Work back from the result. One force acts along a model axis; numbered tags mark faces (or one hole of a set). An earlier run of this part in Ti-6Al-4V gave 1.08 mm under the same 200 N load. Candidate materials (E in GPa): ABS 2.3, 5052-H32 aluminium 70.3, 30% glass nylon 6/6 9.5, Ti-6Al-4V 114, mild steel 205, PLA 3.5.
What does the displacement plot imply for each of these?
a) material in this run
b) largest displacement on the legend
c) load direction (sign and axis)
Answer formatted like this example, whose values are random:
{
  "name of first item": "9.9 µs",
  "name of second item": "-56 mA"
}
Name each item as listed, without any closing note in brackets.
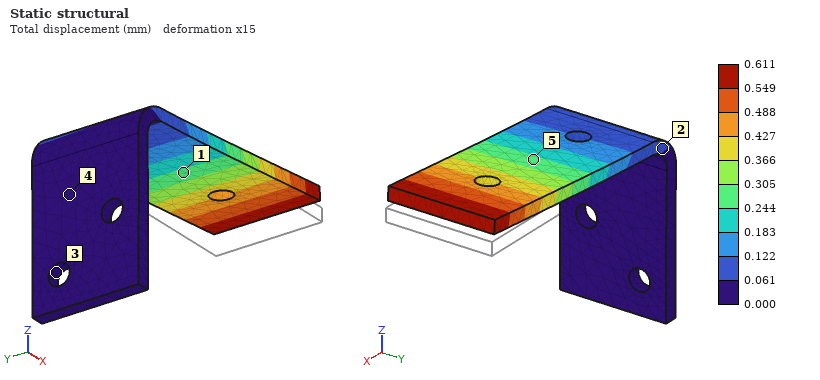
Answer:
{
  "material in this run": "mild steel",
  "largest displacement on the legend": "0.611 mm",
  "load direction": "+Z"
}
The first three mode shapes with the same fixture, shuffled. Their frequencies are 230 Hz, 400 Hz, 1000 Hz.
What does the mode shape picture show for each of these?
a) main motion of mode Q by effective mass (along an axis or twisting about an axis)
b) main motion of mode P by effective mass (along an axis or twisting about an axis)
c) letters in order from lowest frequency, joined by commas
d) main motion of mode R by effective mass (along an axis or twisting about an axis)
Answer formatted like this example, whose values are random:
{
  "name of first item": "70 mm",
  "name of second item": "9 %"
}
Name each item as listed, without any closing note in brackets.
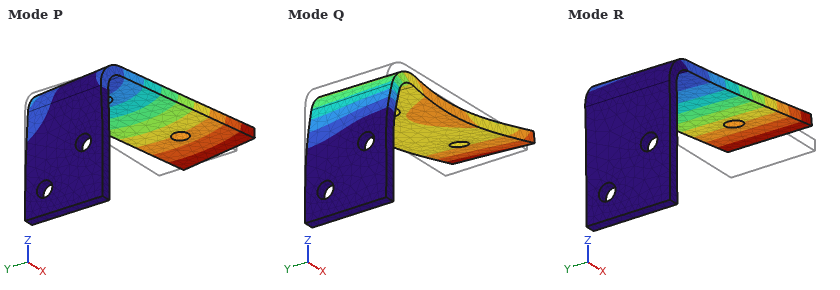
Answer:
{
  "main motion of mode Q by effective mass": "along X",
  "main motion of mode P by effective mass": "along Y",
  "letters in order from lowest frequency, joined by commas": "R, P, Q",
  "main motion of mode R by effective mass": "along Z"
}
